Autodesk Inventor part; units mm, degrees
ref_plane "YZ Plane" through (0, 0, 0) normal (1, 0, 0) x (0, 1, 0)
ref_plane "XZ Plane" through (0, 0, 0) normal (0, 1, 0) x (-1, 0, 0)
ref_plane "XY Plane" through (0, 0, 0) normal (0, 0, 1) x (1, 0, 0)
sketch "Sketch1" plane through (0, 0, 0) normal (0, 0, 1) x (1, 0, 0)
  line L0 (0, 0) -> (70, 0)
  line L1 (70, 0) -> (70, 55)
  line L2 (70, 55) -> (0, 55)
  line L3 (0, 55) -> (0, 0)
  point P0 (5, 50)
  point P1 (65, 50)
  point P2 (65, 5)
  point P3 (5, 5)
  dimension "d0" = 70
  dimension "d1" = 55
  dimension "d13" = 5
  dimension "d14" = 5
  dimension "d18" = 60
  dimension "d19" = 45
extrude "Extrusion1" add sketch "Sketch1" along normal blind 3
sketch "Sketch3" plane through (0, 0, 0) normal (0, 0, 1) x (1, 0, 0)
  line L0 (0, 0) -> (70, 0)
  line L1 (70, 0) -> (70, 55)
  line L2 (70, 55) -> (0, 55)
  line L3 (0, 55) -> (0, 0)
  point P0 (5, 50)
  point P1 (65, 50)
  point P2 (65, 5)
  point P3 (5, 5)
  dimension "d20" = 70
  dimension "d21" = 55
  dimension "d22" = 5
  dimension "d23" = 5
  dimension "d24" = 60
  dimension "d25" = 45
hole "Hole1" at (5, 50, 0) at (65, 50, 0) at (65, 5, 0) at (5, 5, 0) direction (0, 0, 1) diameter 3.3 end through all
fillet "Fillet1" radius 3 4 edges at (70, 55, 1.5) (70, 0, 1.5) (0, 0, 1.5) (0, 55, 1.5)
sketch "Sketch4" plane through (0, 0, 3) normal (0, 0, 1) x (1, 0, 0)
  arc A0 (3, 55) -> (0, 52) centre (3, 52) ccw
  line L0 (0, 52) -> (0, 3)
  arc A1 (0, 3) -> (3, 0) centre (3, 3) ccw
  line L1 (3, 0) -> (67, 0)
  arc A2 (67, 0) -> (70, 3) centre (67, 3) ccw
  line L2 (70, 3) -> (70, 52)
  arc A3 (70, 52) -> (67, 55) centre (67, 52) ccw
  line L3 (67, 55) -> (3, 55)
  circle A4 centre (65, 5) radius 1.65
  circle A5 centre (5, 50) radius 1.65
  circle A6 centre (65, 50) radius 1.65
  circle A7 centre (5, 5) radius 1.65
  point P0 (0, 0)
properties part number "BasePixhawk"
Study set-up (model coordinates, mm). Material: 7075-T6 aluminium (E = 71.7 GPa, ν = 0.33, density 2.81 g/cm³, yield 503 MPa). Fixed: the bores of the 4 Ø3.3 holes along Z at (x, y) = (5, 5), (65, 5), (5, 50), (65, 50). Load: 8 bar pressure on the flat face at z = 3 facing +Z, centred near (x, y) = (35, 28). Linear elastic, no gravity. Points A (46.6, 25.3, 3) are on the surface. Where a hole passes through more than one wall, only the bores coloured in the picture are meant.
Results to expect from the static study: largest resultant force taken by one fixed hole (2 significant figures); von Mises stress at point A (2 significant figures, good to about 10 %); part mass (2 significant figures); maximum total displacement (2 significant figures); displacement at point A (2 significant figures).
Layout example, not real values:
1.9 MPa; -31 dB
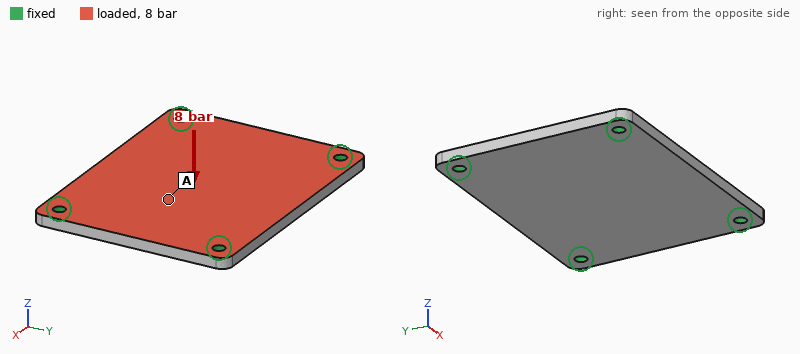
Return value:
760 N; 66 MPa; 32 g; 0.28 mm; 0.24 mm
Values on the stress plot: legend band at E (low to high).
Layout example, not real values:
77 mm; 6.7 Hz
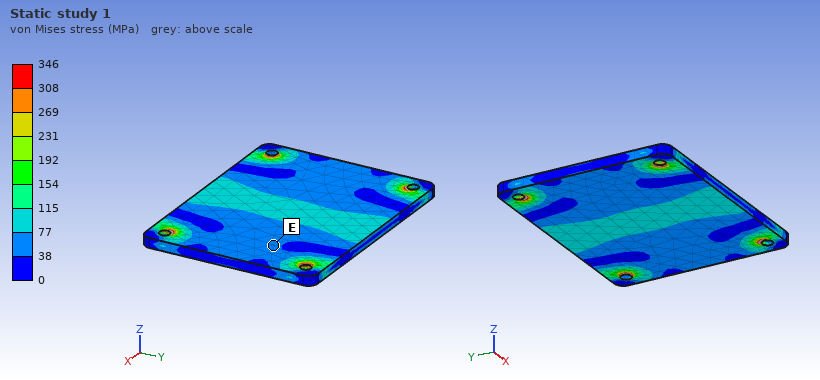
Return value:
38 to 77 MPa
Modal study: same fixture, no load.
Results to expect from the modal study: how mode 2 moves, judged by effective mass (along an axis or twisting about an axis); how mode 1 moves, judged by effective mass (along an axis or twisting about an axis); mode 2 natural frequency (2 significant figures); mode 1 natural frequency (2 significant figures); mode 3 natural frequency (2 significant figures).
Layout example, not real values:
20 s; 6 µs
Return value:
twisting about X; along Z; 5300 Hz; 3500 Hz; 7300 Hz
